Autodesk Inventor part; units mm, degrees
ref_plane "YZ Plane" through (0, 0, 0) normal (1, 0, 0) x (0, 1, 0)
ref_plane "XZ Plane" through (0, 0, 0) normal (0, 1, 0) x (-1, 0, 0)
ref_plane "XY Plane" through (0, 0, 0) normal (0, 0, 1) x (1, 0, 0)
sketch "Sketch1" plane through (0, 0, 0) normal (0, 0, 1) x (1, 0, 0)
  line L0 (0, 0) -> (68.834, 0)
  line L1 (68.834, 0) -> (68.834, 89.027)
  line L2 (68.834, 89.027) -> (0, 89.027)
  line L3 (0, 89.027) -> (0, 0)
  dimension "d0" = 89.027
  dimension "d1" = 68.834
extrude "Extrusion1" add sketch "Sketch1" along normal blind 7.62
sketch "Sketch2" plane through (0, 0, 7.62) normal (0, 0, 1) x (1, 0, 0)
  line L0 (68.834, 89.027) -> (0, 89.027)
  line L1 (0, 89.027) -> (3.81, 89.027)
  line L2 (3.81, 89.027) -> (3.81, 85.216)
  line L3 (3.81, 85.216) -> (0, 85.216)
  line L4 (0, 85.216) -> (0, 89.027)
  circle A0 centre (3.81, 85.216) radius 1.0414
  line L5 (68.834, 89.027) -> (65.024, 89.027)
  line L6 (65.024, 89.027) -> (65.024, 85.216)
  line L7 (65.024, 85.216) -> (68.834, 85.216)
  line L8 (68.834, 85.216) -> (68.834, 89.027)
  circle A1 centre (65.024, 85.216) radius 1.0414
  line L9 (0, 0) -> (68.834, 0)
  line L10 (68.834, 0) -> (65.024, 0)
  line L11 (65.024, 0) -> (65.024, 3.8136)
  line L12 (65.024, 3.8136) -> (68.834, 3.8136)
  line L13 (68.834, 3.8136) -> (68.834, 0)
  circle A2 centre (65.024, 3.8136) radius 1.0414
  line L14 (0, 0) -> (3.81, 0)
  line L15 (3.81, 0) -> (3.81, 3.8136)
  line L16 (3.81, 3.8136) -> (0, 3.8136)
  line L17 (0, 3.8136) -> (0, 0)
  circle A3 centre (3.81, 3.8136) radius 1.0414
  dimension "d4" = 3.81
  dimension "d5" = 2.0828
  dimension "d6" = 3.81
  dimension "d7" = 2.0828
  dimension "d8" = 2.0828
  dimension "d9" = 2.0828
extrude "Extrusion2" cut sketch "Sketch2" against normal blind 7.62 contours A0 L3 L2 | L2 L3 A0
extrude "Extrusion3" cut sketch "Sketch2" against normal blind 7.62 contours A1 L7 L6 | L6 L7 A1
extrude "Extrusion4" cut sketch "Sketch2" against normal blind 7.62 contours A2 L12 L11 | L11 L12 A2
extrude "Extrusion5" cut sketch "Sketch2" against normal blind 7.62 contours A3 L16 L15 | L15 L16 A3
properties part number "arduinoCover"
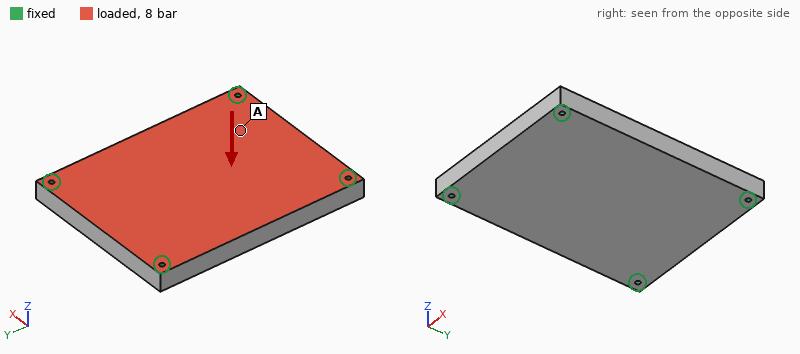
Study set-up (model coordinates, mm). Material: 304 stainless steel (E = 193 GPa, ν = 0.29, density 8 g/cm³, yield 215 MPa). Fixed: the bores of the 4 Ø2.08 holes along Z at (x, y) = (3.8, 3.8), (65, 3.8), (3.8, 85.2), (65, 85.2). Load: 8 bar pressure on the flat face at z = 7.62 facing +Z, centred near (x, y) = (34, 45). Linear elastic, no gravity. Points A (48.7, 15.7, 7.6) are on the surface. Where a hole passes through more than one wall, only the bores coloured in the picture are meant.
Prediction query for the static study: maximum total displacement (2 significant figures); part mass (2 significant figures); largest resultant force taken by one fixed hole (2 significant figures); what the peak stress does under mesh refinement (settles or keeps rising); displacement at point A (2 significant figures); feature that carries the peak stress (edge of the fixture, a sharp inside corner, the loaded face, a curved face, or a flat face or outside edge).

34 µm
370 g
1.2 kN
keeps rising
18 µm
edge of the fixture
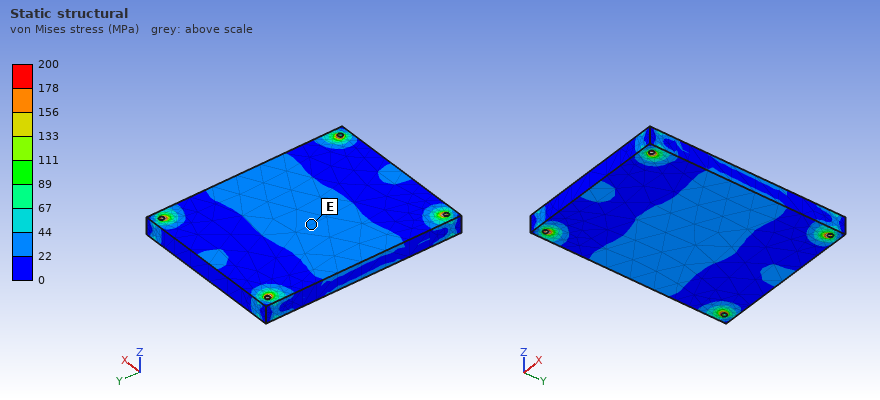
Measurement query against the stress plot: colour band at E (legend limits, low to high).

22 to 44 MPa
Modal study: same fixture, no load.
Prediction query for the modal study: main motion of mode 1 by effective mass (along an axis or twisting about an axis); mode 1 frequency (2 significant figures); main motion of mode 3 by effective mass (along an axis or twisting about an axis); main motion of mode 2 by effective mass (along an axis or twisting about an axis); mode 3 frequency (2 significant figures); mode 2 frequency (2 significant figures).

along Z
3600 Hz
twisting about X
twisting about Y
7900 Hz
6200 Hz
